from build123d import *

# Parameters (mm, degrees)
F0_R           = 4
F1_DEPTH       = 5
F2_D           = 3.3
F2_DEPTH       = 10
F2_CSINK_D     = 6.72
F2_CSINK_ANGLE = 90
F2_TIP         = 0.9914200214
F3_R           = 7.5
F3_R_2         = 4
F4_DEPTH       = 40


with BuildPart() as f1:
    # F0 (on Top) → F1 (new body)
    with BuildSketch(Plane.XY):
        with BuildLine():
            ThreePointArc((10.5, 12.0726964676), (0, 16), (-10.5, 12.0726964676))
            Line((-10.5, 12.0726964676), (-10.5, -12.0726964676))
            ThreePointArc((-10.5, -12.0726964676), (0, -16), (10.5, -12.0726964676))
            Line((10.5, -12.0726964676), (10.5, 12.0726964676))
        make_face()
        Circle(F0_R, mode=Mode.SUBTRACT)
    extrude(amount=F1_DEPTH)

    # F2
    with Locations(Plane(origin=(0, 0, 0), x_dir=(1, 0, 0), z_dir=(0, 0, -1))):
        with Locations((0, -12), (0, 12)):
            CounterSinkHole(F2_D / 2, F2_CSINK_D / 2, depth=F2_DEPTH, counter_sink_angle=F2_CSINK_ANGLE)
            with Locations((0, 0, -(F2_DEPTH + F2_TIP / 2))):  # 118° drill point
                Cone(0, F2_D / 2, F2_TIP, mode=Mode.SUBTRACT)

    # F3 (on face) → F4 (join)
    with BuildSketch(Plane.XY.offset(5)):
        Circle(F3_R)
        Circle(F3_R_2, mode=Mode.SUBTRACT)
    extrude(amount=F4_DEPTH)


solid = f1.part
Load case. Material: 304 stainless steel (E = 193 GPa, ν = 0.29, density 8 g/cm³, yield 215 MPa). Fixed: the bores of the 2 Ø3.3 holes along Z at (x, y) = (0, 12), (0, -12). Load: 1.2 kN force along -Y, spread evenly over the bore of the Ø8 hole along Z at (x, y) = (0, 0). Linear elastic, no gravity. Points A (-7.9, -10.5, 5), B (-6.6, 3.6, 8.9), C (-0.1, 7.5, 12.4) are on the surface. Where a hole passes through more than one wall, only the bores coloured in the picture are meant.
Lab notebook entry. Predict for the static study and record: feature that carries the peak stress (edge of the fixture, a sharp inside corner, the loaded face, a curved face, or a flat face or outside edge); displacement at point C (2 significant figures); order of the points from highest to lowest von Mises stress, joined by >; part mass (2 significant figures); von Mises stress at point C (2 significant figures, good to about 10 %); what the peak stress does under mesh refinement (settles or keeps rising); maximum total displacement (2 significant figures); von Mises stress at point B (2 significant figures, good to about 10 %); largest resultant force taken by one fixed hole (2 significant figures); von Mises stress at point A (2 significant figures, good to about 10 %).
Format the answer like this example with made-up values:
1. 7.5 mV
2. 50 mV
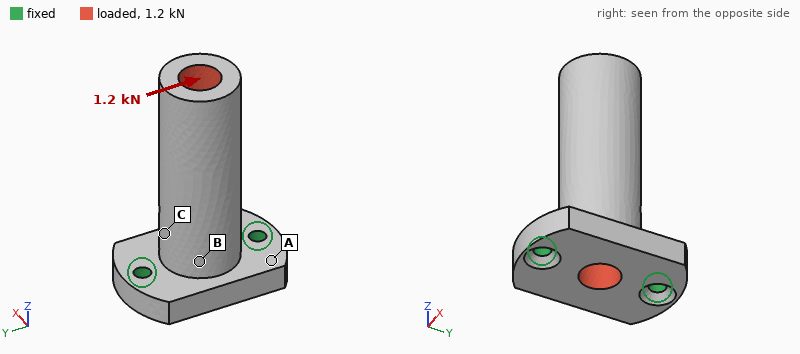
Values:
1. edge of the fixture
2. 8.9 µm
3. C > B > A
4. 62 g
5. 43 MPa
6. keeps rising
7. 43 µm
8. 27 MPa
9. 1.3 kN
10. 14 MPa
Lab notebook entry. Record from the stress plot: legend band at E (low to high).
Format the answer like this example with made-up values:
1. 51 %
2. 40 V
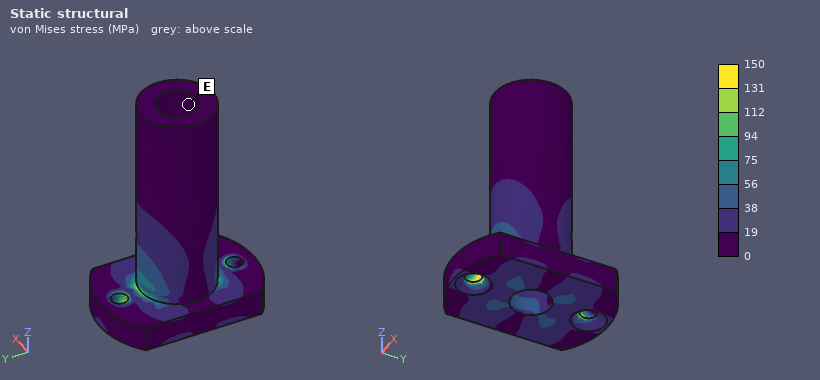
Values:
1. 0 to 19 MPa
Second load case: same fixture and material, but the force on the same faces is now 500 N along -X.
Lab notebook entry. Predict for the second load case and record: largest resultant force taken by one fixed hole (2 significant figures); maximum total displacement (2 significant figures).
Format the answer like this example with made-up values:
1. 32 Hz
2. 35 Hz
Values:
1. 250 N
2. 61 µm
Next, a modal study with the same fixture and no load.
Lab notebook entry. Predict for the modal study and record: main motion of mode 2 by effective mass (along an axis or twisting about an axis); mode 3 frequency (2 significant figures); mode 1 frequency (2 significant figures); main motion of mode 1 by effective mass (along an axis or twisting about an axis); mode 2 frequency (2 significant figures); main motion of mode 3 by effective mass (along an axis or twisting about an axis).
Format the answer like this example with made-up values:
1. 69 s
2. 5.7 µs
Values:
1. along Y
2. 14 kHz
3. 2600 Hz
4. along X
5. 4800 Hz
6. along Z
